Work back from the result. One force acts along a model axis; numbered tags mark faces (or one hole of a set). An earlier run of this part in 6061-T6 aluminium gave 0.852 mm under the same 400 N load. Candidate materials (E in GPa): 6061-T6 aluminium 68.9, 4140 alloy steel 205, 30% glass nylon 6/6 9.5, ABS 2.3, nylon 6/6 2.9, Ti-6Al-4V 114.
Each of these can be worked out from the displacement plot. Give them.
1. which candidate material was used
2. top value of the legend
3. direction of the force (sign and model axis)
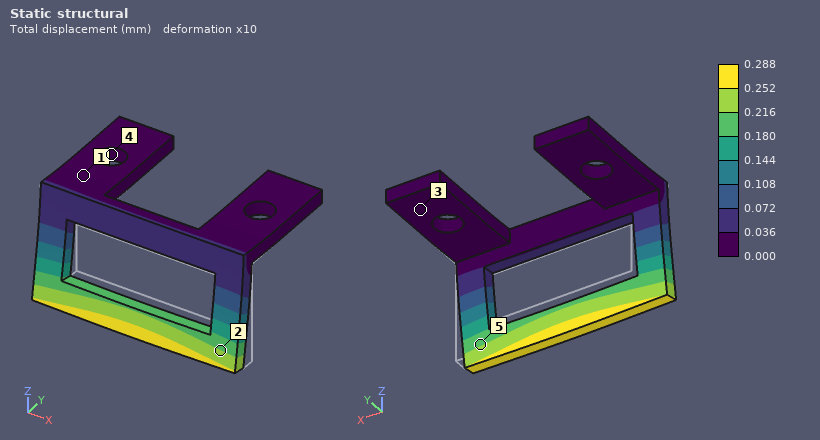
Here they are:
4140 alloy steel
0.288 mm
-Y
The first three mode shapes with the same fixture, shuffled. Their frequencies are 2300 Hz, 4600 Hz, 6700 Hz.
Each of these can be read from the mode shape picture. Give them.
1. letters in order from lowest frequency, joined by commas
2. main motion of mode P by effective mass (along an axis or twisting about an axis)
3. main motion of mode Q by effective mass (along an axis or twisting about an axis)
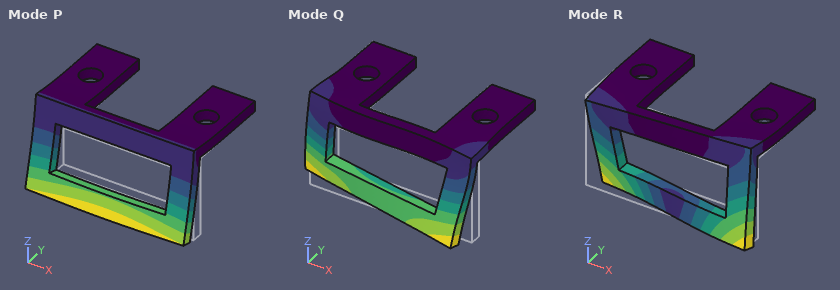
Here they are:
P, R, Q
along Y
along X
